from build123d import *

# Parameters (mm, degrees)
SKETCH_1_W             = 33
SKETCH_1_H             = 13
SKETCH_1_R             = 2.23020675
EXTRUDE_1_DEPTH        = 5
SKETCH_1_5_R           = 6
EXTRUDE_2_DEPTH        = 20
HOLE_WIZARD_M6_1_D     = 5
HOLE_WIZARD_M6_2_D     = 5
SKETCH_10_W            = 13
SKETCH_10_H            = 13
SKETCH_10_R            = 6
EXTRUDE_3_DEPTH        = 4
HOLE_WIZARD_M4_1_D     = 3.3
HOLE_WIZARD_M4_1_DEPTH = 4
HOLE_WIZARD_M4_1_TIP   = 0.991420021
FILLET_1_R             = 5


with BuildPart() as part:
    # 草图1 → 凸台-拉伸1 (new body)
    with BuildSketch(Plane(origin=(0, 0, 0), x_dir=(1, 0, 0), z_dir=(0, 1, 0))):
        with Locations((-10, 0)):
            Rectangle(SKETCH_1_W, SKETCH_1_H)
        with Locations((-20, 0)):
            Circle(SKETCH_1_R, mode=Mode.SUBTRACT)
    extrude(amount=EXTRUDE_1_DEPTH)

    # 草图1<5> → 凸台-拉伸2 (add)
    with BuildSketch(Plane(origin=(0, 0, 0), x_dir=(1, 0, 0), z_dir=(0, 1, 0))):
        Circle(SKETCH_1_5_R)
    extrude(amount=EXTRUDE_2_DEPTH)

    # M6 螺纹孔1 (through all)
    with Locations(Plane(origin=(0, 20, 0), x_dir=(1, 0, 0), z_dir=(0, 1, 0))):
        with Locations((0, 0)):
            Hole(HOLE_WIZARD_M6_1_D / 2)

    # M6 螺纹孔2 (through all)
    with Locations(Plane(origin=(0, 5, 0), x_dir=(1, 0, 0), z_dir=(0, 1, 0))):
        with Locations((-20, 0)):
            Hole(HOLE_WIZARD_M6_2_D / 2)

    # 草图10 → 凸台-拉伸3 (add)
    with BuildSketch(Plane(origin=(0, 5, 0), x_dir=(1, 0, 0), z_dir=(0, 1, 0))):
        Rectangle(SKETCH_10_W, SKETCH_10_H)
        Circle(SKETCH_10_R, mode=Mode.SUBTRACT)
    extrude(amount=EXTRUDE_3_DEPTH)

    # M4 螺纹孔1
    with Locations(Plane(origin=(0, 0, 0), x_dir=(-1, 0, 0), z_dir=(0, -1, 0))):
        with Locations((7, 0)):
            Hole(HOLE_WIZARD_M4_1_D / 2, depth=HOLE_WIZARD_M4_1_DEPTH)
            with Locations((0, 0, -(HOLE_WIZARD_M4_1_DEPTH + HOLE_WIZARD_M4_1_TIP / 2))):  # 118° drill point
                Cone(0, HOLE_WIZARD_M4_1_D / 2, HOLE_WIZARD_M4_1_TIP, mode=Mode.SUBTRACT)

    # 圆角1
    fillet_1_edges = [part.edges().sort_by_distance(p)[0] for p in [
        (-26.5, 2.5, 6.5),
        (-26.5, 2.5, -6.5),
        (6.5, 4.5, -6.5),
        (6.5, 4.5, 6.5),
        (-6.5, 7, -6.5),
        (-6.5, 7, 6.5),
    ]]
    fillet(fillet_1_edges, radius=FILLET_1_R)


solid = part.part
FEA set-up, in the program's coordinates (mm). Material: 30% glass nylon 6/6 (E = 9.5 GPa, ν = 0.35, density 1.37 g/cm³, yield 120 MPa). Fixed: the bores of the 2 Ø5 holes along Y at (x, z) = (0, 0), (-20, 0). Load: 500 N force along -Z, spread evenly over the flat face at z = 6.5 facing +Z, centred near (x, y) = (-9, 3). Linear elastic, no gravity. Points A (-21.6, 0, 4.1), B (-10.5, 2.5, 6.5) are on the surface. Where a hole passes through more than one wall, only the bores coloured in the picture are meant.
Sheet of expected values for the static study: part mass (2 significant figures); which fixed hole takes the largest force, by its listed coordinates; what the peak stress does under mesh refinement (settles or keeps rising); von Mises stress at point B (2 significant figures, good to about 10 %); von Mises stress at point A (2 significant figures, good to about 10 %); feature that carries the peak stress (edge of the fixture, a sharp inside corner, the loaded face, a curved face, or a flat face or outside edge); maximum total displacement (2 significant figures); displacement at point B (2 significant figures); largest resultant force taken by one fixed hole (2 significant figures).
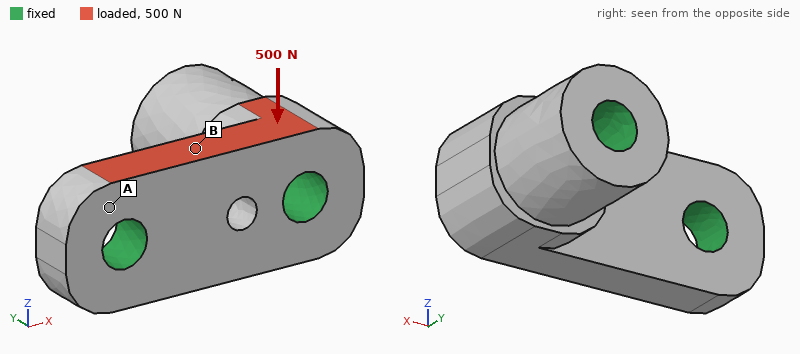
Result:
4.6 g
(0, 0)
keeps rising
4.9 MPa
1.4 MPa
edge of the fixture
7.2 µm
6.3 µm
280 N
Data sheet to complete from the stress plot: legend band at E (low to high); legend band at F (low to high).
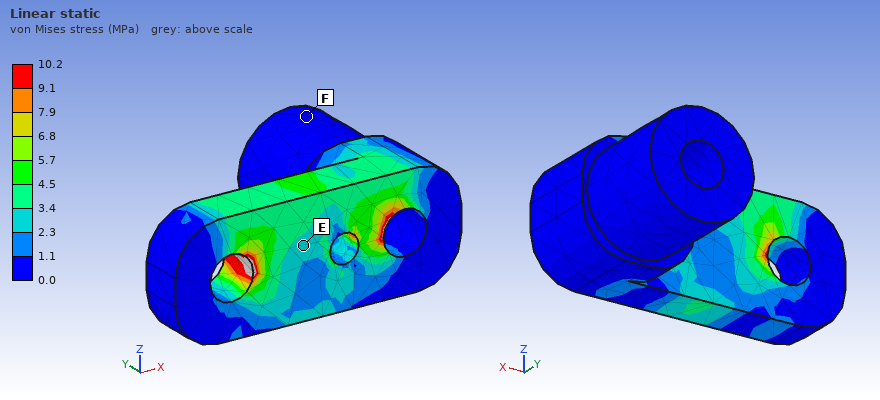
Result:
2.3 to 3.4 MPa
0.0 to 1.1 MPa
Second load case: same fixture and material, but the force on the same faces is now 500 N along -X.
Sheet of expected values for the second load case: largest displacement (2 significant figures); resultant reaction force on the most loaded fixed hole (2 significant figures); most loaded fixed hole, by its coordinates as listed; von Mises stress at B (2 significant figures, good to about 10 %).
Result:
6.3 µm
290 N
(0, 0)
6.8 MPa
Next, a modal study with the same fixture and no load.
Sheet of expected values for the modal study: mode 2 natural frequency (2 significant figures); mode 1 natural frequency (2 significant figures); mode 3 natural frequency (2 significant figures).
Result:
36 kHz
35 kHz
39 kHz
